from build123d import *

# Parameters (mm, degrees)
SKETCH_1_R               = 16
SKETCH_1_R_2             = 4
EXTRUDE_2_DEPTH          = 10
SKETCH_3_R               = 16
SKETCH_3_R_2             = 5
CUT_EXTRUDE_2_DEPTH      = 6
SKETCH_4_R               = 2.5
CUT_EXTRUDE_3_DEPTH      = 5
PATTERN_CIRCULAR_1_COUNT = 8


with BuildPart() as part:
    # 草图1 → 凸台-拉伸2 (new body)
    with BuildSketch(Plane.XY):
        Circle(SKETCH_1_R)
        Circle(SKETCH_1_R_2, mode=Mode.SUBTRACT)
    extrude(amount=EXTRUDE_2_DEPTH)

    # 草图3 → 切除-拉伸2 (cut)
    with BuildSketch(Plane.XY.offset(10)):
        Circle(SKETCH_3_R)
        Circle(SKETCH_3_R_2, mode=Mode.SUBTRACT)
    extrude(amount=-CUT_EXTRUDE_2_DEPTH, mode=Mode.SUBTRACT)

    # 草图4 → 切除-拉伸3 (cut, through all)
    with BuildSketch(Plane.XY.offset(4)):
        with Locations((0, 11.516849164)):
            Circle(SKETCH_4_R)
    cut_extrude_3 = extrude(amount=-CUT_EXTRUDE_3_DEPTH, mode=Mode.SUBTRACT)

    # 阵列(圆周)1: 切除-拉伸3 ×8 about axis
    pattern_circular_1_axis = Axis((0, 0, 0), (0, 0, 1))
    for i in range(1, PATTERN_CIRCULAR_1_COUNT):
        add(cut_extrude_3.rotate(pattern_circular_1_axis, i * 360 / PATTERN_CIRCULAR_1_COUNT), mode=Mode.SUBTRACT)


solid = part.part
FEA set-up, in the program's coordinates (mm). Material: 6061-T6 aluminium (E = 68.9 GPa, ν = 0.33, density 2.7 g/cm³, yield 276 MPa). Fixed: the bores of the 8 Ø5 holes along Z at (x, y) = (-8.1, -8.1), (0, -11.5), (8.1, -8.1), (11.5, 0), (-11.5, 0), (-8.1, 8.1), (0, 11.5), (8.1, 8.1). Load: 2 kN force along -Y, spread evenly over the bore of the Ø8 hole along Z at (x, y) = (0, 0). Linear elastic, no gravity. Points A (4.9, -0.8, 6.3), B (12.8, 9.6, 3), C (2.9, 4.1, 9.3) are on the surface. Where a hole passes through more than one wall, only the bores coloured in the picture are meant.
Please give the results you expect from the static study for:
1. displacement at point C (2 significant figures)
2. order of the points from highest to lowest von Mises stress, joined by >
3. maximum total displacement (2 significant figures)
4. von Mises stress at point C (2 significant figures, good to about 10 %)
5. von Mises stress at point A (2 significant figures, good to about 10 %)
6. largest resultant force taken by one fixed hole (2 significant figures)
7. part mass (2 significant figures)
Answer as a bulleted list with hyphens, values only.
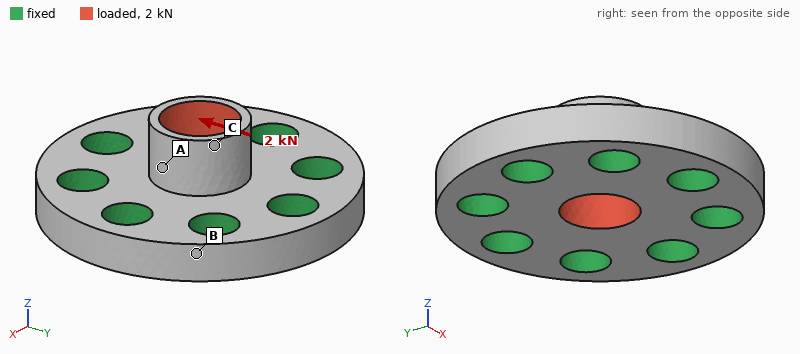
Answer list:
- 18 µm
- A > C > B
- 20 µm
- 34 MPa
- 67 MPa
- 470 N
- 6.9 g
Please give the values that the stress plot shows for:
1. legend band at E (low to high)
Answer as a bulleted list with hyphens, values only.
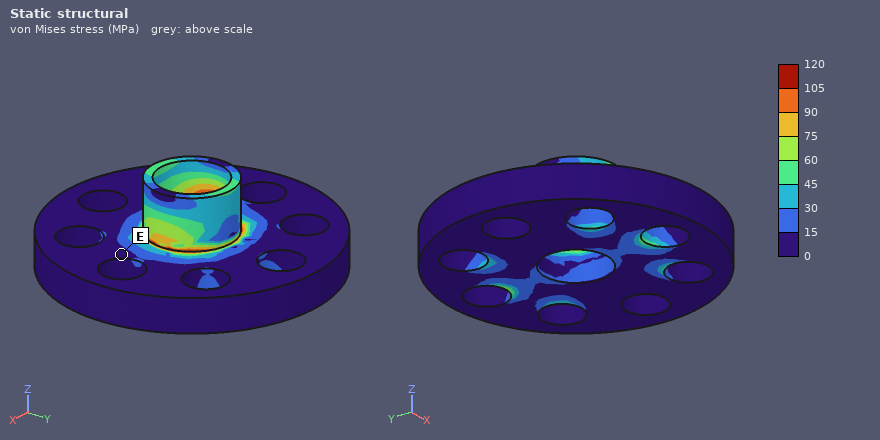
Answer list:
- 0 to 15 MPa
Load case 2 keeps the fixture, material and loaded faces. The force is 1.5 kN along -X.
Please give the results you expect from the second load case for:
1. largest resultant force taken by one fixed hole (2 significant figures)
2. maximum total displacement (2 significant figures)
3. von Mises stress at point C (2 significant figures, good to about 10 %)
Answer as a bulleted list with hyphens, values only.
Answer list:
- 360 N
- 15 µm
- 19 MPa
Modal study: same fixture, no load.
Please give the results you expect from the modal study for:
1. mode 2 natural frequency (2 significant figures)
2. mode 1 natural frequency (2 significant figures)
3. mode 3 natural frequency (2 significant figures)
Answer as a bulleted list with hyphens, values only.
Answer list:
- 58 kHz
- 58 kHz
- 66 kHz
